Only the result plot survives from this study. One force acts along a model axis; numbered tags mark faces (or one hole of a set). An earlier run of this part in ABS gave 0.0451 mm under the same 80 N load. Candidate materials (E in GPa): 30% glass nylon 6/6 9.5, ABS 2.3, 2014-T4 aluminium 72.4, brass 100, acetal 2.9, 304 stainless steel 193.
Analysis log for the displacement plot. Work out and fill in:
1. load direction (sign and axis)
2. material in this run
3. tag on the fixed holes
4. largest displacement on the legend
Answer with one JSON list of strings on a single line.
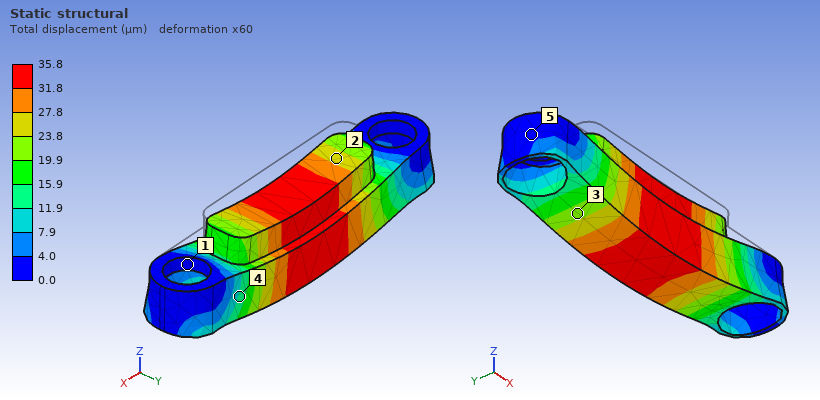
["-Z", "acetal", "1", "35.8 µm"]
